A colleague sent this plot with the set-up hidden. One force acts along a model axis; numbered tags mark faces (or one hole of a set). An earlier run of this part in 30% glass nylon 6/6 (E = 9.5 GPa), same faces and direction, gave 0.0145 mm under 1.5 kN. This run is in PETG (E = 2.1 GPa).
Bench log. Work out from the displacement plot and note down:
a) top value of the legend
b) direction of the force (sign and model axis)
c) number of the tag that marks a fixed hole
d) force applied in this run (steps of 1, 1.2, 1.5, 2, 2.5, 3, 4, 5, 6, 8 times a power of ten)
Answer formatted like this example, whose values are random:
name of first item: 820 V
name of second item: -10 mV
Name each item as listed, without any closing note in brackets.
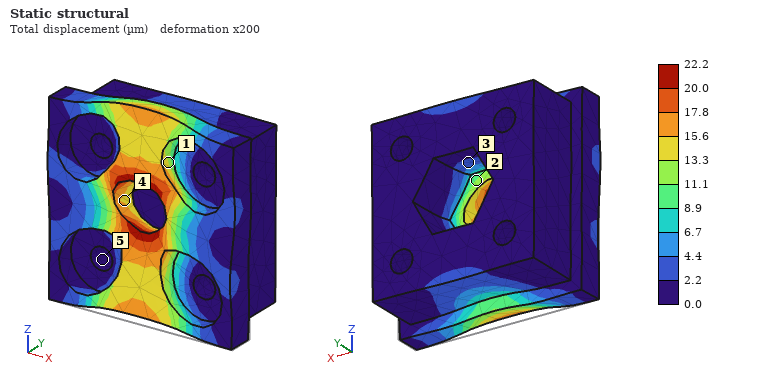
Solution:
top value of the legend: 22.2 µm
direction of the force: +Z
number of the tag that marks a fixed hole: 5
force applied in this run: 500 N
